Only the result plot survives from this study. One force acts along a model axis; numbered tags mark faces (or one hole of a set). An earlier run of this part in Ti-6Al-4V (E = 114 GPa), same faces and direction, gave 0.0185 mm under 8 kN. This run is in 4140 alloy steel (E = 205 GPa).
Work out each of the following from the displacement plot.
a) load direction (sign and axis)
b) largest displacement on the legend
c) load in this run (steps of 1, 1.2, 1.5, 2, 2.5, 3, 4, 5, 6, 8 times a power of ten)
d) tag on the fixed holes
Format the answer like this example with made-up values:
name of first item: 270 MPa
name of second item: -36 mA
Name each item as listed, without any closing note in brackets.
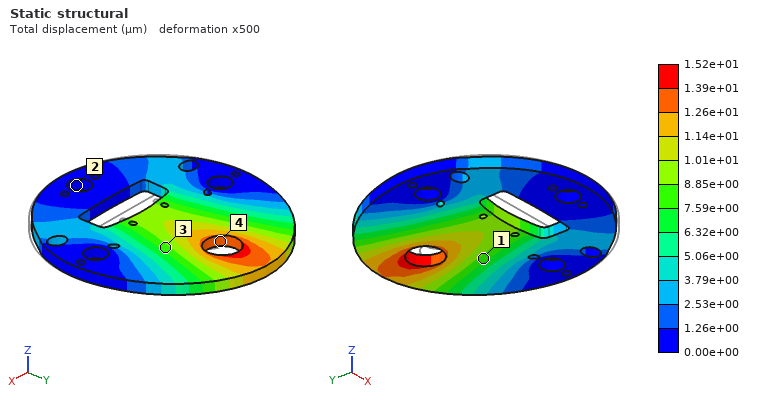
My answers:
load direction: +Y
largest displacement on the legend: 1.52e+01 µm
load in this run: 12 kN
tag on the fixed holes: 2
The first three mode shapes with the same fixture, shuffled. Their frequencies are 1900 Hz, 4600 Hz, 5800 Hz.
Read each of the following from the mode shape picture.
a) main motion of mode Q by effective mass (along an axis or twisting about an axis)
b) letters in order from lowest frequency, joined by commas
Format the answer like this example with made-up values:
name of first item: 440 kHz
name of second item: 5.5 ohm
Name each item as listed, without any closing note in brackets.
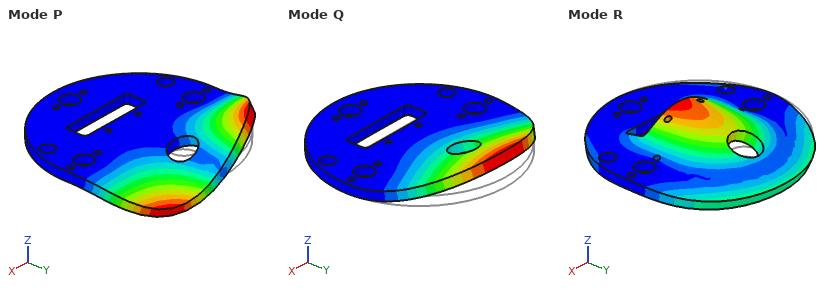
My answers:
main motion of mode Q by effective mass: along Z
letters in order from lowest frequency, joined by commas: Q, P, R
